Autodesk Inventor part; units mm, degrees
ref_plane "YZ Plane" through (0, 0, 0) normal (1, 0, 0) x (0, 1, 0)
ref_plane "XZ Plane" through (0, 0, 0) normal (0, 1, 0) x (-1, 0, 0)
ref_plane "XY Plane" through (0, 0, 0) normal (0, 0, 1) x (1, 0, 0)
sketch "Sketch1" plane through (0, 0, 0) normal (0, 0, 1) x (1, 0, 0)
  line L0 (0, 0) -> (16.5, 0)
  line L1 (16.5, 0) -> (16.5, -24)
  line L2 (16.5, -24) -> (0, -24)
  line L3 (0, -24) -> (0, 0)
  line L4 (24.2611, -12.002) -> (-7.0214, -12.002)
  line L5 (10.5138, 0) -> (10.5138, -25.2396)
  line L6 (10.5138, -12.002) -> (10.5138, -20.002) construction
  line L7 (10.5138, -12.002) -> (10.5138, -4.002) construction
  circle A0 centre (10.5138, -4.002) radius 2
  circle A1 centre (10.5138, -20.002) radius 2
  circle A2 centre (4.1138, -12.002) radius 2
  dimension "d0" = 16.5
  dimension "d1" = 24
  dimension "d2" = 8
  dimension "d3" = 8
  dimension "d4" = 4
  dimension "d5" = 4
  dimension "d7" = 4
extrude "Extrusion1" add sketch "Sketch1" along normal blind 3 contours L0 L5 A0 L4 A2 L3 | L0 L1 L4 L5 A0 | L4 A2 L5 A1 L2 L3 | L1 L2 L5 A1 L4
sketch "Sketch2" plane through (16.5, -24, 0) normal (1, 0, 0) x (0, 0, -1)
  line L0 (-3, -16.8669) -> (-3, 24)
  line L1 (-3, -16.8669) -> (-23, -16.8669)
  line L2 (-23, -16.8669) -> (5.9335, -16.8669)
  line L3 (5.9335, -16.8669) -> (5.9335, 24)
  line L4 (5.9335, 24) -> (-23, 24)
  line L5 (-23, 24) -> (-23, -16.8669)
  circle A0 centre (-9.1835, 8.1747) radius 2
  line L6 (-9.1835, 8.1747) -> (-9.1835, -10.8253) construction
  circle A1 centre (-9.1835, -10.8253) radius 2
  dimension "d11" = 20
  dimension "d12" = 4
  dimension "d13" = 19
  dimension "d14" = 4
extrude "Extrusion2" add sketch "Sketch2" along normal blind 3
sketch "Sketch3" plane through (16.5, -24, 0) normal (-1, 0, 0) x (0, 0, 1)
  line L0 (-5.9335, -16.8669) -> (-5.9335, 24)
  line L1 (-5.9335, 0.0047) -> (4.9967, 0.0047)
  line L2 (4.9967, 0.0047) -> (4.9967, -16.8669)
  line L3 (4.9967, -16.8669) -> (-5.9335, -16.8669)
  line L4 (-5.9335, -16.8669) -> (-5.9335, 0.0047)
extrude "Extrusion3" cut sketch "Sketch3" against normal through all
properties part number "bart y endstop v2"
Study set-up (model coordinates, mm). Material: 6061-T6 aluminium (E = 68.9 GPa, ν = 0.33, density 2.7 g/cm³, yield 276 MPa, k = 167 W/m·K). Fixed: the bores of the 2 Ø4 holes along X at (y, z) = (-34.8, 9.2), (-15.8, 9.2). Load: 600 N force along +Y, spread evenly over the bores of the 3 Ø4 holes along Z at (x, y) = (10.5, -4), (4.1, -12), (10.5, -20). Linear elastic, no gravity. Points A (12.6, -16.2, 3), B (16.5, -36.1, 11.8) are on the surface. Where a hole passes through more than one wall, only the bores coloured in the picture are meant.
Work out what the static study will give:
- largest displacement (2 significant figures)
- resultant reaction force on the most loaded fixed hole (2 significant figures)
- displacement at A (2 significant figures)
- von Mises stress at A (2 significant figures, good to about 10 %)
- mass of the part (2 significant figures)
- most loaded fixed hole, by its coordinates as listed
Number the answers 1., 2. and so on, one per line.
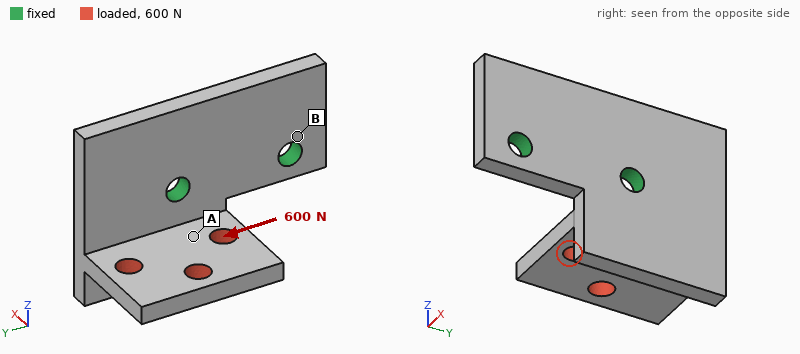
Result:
1. 0.14 mm
2. 610 N
3. 0.035 mm
4. 40 MPa
5. 11 g
6. (-15.8, 9.2)
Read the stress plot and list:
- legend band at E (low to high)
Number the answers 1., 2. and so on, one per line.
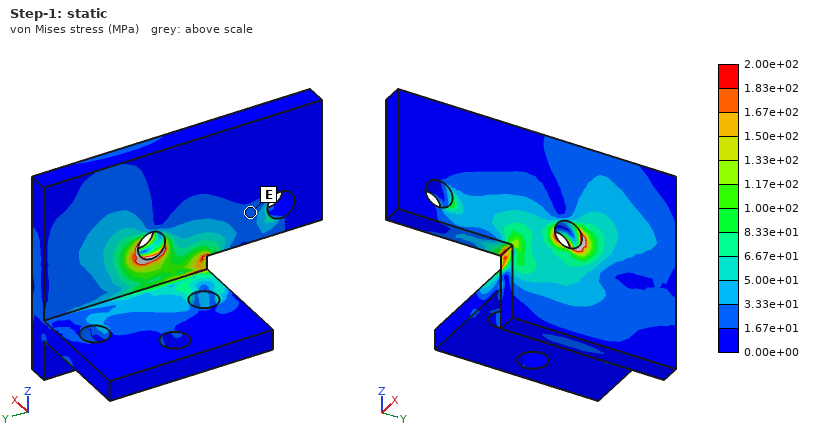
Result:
1. 1.67e+01 to 3.33e+01 MPa
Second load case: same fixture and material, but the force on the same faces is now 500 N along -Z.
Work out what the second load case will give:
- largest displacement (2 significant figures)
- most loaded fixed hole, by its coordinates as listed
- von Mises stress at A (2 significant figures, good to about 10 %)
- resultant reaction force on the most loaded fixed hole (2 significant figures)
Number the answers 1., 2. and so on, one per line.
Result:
1. 0.28 mm
2. (-15.8, 9.2)
3. 70 MPa
4. 560 N
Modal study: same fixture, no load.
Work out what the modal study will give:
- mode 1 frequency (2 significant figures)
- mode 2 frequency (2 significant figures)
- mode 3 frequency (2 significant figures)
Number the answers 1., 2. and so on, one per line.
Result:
1. 4300 Hz
2. 6100 Hz
3. 10 kHz
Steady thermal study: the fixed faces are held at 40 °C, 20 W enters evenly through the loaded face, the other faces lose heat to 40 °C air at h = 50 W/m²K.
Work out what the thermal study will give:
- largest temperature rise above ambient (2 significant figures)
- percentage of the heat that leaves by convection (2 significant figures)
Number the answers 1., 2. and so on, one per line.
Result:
1. 33 K
2. 9.2 %
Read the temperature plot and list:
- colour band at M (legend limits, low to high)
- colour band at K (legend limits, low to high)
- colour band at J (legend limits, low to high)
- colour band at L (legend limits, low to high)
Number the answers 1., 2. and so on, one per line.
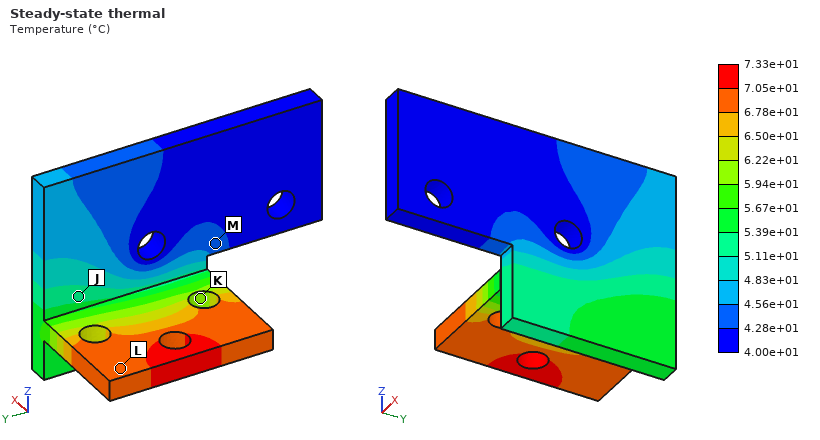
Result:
1. 4.28e+01 to 4.56e+01 °C
2. 5.94e+01 to 6.22e+01 °C
3. 5.11e+01 to 5.39e+01 °C
4. 6.78e+01 to 7.05e+01 °C
